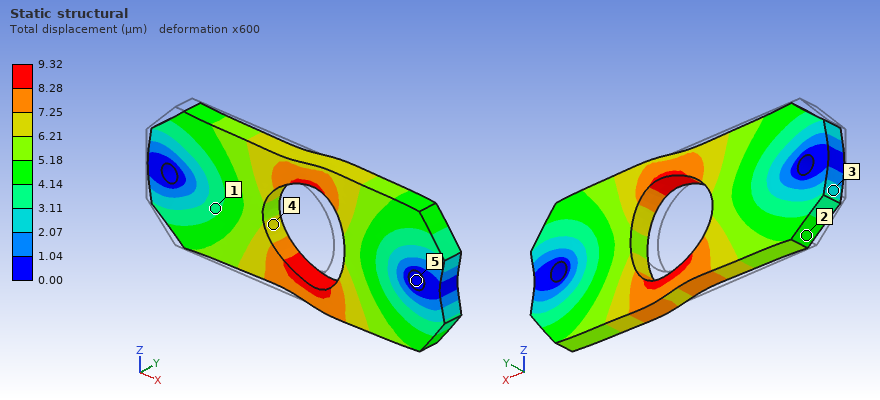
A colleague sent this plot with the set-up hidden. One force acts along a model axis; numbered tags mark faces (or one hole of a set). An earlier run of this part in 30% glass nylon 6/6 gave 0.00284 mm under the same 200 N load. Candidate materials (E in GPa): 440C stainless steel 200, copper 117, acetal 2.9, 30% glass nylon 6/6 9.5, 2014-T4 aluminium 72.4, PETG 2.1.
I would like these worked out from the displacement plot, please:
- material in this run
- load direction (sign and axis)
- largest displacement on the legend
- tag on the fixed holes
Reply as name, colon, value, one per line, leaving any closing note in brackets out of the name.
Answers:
material in this run: acetal
load direction: +X
largest displacement on the legend: 9.32 µm
tag on the fixed holes: 5
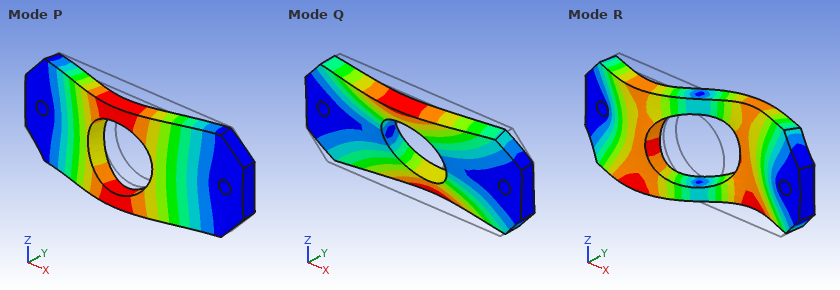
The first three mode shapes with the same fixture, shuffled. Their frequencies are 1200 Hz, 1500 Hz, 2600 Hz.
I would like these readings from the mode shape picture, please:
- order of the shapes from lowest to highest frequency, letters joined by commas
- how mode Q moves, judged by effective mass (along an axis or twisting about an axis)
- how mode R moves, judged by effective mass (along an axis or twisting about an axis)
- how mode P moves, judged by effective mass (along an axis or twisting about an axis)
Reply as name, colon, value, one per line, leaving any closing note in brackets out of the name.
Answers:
order of the shapes from lowest to highest frequency, letters joined by commas: P, Q, R
how mode Q moves, judged by effective mass: twisting about X
how mode R moves, judged by effective mass: twisting about Z
how mode P moves, judged by effective mass: along Y
